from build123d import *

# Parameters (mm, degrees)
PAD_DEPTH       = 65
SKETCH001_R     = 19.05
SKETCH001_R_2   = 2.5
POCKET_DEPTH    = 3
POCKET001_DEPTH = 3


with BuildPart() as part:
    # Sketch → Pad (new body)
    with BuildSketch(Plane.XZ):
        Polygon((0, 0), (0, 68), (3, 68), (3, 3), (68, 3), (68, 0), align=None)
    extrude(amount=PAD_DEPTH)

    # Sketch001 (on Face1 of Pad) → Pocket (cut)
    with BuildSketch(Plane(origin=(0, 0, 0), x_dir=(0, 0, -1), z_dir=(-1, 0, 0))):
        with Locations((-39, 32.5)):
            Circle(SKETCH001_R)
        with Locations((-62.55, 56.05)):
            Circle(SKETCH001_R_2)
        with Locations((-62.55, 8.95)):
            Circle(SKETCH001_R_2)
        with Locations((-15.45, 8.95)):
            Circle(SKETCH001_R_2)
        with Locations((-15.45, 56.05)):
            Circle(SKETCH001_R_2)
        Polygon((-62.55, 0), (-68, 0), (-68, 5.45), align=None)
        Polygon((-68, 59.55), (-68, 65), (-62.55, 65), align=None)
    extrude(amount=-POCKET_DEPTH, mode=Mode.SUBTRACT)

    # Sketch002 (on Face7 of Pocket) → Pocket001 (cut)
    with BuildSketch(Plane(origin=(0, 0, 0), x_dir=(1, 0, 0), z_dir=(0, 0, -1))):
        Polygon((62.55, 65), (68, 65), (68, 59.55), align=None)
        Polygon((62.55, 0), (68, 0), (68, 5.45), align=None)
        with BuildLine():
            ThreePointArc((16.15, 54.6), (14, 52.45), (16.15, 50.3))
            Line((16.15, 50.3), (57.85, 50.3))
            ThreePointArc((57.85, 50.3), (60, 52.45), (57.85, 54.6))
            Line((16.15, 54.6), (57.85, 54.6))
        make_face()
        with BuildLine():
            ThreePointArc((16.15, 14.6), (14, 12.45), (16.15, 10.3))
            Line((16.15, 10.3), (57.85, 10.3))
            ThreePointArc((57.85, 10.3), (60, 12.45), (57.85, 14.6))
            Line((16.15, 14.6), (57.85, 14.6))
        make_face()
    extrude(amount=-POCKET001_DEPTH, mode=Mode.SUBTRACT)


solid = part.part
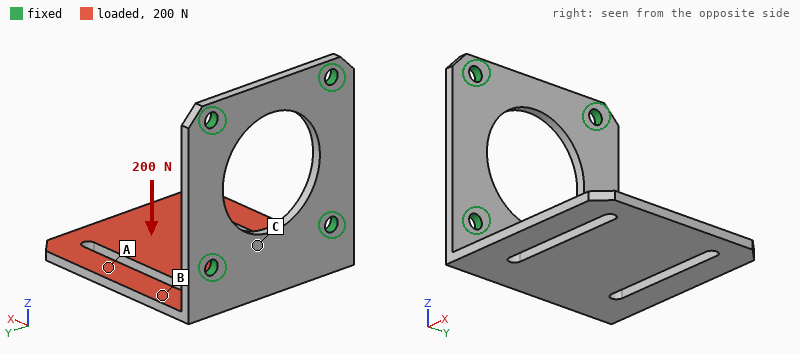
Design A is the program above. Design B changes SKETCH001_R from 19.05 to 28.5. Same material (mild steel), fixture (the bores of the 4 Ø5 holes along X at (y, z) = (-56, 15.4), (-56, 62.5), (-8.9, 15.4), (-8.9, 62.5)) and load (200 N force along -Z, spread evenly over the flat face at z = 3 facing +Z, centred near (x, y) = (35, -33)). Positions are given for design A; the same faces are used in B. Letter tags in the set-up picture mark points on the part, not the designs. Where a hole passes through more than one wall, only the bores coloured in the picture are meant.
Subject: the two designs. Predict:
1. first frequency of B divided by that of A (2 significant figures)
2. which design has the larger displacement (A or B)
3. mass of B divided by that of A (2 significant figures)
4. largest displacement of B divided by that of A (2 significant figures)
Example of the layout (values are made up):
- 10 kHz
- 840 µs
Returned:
- 0.94
- B
- 0.80
- 1.1
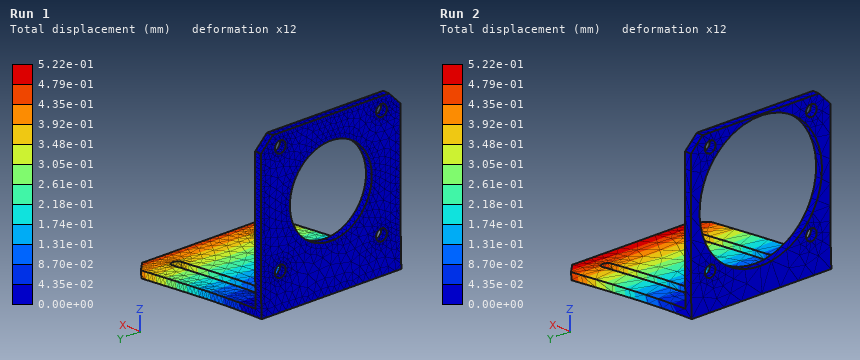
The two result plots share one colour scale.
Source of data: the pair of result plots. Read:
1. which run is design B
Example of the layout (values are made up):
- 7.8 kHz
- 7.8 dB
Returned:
- Run 2
